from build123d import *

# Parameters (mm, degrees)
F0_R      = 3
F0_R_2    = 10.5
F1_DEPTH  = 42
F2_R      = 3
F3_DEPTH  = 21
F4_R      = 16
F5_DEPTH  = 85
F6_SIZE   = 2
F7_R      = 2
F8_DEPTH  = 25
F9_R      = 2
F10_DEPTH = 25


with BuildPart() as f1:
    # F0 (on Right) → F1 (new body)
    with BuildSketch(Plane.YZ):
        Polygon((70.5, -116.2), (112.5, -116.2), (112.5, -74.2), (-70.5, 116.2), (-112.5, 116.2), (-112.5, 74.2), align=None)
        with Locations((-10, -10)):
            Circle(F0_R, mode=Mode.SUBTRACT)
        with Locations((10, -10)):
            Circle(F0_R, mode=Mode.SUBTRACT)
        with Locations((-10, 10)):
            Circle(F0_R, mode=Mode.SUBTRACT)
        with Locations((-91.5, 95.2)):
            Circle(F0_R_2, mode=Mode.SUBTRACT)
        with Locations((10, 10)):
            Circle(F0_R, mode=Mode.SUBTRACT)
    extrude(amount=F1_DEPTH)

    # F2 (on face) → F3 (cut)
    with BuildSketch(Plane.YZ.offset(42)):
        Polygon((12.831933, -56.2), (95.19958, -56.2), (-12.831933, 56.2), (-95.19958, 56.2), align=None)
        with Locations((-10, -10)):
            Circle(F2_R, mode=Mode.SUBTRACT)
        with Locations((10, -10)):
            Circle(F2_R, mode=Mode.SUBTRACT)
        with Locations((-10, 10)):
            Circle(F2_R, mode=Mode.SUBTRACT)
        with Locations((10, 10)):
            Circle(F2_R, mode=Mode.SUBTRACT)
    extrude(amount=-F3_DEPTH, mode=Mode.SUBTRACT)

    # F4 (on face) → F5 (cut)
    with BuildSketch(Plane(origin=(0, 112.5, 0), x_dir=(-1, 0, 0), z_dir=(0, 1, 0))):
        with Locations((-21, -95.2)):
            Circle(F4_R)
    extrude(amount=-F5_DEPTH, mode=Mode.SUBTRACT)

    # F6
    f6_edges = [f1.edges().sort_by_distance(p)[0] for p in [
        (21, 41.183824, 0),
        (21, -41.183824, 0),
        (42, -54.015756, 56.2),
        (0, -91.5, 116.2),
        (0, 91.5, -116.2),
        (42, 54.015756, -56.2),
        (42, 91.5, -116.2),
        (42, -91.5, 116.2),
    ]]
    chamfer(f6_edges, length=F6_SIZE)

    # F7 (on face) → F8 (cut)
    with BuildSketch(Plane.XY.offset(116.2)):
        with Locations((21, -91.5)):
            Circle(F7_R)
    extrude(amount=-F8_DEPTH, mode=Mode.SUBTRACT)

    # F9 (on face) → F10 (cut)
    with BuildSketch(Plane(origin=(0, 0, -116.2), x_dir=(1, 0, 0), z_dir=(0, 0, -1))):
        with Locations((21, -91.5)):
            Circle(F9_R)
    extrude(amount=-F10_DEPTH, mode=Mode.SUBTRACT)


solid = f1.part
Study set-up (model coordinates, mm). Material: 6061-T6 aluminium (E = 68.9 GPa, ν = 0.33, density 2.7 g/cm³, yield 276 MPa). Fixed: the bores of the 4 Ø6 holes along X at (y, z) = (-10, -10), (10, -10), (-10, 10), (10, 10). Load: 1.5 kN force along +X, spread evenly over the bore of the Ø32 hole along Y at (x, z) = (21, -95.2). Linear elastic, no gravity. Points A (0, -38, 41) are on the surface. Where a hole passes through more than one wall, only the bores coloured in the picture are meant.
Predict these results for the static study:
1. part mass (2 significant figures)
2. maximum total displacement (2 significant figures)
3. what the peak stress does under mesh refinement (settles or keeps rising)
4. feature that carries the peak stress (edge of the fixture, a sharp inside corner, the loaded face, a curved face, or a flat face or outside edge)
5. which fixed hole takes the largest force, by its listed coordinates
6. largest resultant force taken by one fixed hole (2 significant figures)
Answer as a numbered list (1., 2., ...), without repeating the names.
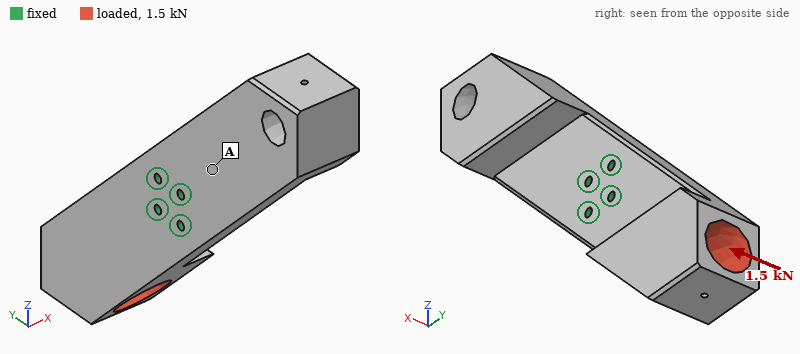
1. 1.3 kg
2. 0.34 mm
3. keeps rising
4. edge of the fixture
5. (10, -10)
6. 3.9 kN
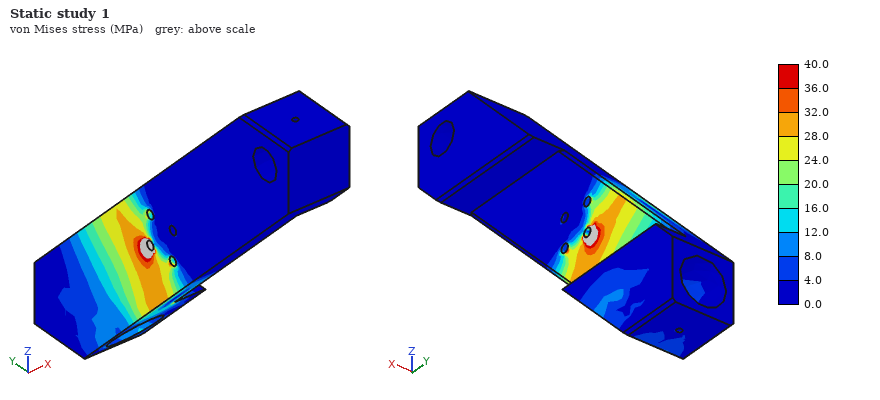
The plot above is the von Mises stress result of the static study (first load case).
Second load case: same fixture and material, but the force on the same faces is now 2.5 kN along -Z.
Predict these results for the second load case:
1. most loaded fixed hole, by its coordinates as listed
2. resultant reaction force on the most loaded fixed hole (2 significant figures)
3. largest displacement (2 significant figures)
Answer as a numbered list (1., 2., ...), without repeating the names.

1. (10, 10)
2. 4.4 kN
3. 0.10 mm
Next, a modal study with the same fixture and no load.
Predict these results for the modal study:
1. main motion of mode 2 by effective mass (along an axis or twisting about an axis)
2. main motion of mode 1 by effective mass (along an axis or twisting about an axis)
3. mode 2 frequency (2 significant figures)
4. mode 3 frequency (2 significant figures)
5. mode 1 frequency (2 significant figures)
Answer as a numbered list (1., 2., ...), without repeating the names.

1. along X
2. along X
3. 800 Hz
4. 1400 Hz
5. 690 Hz
